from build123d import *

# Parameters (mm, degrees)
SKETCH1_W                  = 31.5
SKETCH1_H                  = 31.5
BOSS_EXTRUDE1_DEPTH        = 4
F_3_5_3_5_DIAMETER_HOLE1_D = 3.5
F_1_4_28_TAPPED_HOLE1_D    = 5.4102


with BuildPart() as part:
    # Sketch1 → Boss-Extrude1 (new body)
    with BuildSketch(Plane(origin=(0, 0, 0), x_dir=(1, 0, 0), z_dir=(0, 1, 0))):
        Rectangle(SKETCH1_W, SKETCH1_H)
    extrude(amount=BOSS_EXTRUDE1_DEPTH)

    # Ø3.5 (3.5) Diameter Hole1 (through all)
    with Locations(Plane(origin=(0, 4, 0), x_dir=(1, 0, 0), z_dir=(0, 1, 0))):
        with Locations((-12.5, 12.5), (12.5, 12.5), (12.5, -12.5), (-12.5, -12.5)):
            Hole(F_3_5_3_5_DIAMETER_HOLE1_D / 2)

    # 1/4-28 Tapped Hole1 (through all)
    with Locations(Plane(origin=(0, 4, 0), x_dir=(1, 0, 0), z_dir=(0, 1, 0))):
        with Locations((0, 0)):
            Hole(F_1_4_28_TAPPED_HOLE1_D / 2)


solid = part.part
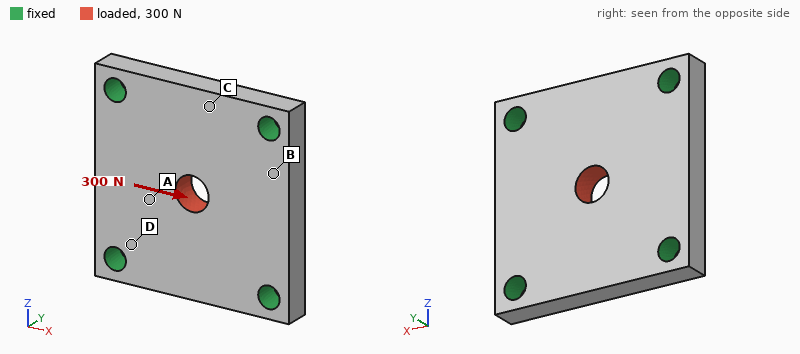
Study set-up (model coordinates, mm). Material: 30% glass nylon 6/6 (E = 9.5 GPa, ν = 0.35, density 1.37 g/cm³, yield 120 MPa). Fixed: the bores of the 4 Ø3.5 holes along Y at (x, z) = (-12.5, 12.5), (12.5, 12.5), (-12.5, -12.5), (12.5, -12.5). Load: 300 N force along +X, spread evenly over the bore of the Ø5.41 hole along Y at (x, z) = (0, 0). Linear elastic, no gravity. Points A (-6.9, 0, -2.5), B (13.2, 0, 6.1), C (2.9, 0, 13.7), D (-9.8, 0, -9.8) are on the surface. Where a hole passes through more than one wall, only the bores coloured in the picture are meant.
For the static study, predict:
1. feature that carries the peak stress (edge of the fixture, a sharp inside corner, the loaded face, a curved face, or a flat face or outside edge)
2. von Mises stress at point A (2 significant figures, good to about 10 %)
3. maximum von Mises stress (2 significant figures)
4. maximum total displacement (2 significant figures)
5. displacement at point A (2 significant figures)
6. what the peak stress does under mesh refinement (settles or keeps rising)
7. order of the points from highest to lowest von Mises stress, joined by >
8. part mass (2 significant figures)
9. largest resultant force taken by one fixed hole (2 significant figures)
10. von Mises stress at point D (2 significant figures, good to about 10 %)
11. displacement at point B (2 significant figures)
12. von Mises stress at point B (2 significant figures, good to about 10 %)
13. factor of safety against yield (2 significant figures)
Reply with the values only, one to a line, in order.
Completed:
the loaded face
2.4 MPa
7.6 MPa
5.9 µm
4.1 µm
settles
D > A > B > C
5.1 g
85 N
3.3 MPa
2.5 µm
1.3 MPa
16
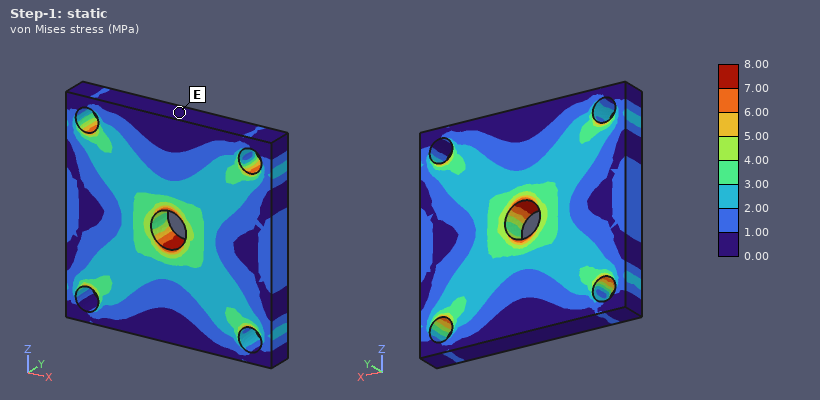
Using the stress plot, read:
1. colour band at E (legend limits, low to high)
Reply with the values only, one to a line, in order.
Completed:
0.00 to 1.00 MPa
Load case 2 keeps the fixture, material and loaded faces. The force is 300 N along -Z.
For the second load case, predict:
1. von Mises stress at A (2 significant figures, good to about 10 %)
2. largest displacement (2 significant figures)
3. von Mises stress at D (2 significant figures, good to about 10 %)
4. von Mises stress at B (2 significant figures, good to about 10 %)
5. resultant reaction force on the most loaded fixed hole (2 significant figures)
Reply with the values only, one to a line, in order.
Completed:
2.2 MPa
5.9 µm
3.3 MPa
1.1 MPa
85 N
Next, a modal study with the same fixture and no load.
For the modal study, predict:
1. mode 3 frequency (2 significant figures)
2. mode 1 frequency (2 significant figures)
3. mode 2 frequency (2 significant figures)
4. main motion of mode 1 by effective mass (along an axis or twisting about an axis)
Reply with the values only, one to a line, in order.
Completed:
18 kHz
12 kHz
18 kHz
along Y
